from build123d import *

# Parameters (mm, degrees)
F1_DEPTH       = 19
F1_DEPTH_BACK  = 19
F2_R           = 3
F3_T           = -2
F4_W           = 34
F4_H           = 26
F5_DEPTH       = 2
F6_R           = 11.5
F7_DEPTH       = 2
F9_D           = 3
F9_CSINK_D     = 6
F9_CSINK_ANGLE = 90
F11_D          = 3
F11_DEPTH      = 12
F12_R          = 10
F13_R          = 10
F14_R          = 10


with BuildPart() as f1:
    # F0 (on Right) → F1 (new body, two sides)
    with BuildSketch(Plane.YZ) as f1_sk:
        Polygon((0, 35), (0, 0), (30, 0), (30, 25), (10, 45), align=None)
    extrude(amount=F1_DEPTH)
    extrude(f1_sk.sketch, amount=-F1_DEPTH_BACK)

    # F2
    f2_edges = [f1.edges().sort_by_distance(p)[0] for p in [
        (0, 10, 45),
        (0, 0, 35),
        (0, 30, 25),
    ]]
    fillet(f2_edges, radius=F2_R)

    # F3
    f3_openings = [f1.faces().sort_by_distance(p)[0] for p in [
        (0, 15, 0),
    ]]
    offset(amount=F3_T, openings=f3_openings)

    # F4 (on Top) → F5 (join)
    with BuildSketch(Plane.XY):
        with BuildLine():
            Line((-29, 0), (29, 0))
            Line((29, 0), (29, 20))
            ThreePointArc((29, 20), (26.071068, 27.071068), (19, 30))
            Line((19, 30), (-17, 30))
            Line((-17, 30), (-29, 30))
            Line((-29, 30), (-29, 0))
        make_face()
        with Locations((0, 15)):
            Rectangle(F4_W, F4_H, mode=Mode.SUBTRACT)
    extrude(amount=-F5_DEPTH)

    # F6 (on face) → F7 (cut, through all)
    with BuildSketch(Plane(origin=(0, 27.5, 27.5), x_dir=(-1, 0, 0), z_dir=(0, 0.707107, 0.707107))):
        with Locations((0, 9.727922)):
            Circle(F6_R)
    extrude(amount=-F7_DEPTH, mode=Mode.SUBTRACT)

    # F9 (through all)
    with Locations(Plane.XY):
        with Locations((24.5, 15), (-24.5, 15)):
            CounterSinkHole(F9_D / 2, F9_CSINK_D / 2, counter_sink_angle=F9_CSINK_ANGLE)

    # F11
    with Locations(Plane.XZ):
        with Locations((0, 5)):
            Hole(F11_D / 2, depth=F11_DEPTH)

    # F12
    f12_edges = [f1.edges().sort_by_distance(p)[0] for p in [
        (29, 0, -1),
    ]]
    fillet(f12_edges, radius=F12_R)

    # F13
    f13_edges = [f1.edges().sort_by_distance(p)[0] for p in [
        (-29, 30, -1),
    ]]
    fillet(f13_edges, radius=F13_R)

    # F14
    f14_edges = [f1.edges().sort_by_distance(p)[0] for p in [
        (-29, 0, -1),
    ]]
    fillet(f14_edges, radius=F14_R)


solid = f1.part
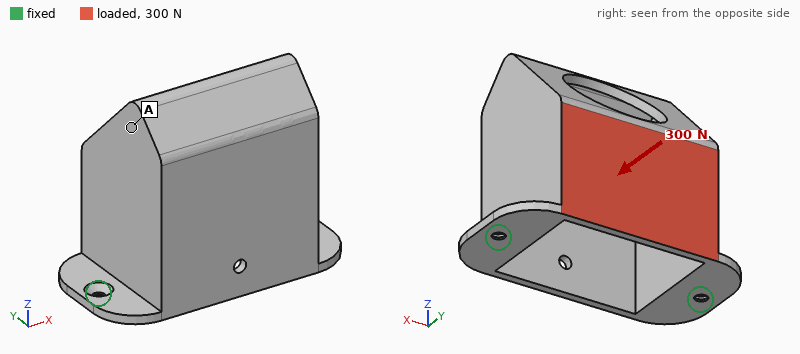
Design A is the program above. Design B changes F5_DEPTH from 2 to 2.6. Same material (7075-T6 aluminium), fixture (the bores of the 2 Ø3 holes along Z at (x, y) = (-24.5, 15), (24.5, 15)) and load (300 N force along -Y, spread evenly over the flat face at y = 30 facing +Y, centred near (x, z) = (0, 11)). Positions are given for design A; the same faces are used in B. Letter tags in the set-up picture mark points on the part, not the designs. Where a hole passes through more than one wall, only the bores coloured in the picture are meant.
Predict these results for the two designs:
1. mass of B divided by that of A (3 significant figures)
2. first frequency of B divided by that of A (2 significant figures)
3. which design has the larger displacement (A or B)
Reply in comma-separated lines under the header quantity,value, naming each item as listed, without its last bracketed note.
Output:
quantity,value
mass of B divided by that of A,1.04
first frequency of B divided by that of A,1.6
which design has the larger displacement,A
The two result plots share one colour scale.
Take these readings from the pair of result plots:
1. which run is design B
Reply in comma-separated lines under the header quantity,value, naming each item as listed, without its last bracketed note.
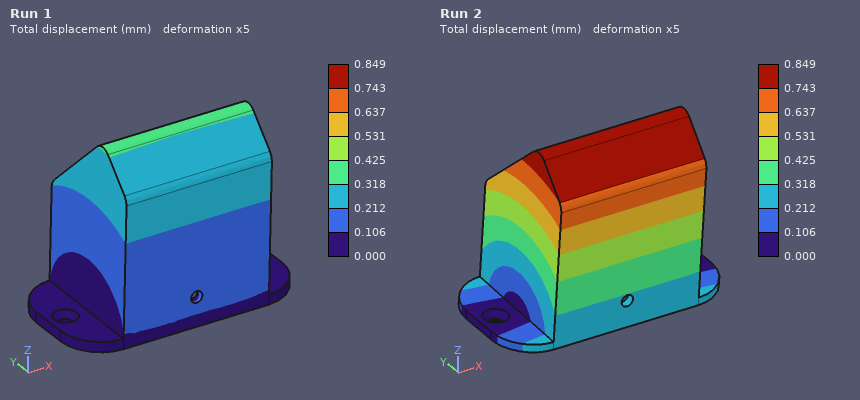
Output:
quantity,value
which run is design B,Run 1
